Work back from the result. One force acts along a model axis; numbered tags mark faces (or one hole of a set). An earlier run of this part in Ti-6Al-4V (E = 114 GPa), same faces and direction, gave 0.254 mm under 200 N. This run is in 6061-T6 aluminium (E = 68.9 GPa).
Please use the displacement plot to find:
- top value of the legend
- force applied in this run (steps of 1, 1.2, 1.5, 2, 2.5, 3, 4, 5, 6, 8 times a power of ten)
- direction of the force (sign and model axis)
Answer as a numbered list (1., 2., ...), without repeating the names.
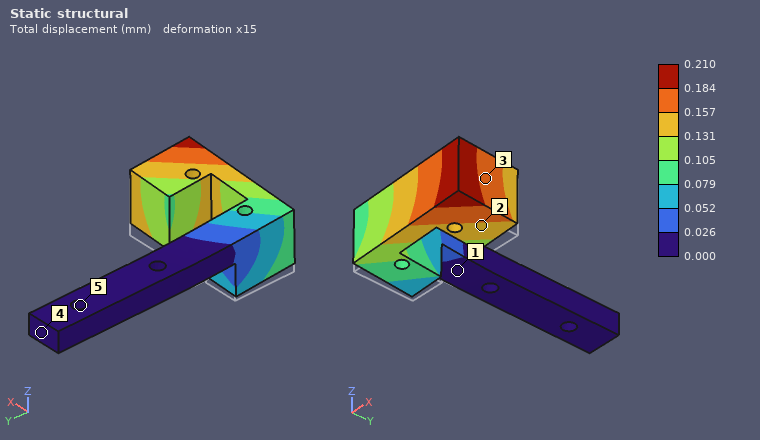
1. 0.210 mm
2. 100 N
3. +Z
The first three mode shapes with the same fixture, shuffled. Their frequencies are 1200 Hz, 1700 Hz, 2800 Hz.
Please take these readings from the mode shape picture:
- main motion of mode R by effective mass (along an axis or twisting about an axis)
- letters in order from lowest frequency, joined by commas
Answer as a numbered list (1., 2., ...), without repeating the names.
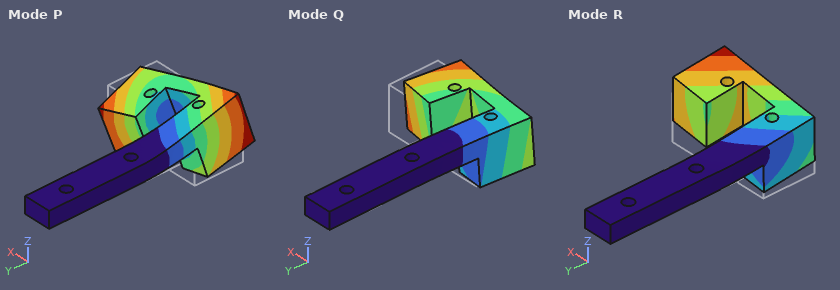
1. along Z
2. R, Q, P
